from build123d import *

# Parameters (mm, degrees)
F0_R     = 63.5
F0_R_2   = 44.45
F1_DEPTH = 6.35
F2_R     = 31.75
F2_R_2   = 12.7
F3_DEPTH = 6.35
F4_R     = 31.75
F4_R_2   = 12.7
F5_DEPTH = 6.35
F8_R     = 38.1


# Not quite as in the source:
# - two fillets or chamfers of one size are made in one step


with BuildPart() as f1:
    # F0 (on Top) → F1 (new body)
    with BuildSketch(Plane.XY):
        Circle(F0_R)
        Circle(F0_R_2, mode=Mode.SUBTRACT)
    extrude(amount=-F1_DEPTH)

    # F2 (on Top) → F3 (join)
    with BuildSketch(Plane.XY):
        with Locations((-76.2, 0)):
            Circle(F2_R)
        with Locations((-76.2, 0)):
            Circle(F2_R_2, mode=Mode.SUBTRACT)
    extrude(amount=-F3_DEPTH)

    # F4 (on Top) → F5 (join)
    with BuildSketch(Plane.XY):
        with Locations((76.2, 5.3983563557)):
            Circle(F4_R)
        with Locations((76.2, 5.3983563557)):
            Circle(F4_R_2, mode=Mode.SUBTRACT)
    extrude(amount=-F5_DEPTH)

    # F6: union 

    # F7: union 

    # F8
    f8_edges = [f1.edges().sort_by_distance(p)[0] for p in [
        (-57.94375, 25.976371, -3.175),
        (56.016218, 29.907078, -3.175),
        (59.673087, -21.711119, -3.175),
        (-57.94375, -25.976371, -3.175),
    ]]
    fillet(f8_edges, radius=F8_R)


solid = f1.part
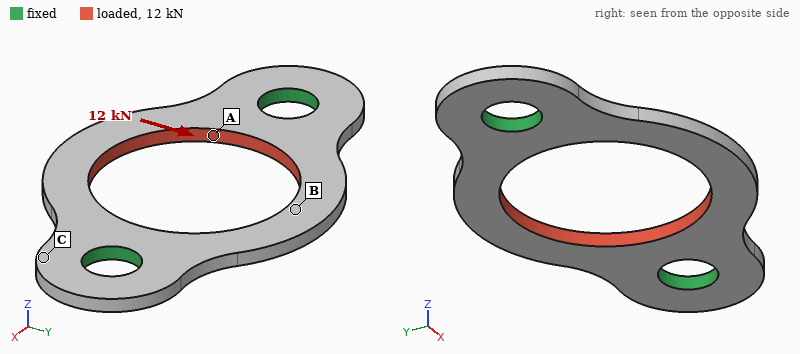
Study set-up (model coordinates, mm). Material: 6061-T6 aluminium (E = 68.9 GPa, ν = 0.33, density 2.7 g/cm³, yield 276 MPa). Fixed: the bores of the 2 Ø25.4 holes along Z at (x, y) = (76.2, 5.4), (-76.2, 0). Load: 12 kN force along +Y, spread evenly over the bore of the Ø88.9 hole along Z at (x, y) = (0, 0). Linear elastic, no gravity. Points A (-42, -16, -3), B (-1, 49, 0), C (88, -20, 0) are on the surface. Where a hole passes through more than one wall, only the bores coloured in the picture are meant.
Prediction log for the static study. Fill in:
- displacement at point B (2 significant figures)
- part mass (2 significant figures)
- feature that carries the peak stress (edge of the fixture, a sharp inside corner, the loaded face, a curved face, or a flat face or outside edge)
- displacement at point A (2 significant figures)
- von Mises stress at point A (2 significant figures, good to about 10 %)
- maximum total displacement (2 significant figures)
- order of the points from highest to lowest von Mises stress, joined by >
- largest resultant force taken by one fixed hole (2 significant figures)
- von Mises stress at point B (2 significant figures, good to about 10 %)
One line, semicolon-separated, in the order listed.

37 µm; 180 g; edge of the fixture; 18 µm; 27 MPa; 38 µm; A > B > C; 6.0 kN; 16 MPa
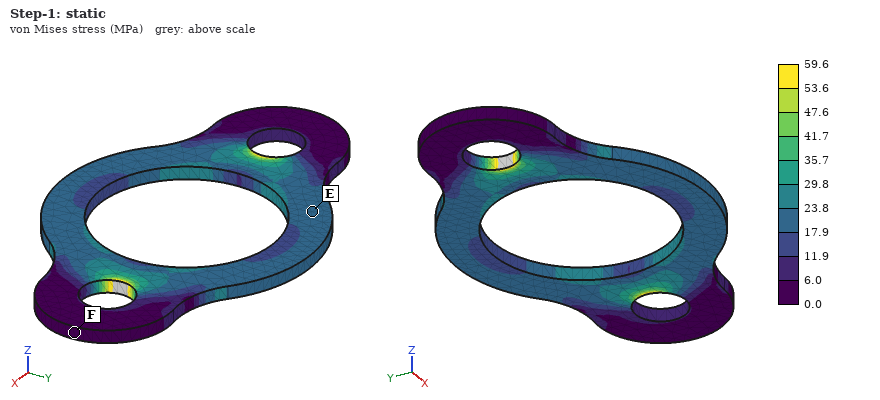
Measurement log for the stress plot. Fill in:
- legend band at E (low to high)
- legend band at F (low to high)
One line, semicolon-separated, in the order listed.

17.9 to 23.8 MPa; 0.0 to 6.0 MPa
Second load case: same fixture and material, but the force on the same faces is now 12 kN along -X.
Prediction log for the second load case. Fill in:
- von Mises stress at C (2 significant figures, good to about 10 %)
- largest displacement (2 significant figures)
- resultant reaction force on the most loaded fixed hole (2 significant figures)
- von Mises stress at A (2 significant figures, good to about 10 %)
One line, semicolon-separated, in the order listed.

8.8 MPa; 37 µm; 6.0 kN; 19 MPa
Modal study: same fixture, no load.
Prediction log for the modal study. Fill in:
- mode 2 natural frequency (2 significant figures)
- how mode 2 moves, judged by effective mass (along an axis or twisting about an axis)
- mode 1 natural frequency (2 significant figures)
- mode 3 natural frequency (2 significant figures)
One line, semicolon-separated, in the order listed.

1300 Hz; along Z; 1100 Hz; 3100 Hz
